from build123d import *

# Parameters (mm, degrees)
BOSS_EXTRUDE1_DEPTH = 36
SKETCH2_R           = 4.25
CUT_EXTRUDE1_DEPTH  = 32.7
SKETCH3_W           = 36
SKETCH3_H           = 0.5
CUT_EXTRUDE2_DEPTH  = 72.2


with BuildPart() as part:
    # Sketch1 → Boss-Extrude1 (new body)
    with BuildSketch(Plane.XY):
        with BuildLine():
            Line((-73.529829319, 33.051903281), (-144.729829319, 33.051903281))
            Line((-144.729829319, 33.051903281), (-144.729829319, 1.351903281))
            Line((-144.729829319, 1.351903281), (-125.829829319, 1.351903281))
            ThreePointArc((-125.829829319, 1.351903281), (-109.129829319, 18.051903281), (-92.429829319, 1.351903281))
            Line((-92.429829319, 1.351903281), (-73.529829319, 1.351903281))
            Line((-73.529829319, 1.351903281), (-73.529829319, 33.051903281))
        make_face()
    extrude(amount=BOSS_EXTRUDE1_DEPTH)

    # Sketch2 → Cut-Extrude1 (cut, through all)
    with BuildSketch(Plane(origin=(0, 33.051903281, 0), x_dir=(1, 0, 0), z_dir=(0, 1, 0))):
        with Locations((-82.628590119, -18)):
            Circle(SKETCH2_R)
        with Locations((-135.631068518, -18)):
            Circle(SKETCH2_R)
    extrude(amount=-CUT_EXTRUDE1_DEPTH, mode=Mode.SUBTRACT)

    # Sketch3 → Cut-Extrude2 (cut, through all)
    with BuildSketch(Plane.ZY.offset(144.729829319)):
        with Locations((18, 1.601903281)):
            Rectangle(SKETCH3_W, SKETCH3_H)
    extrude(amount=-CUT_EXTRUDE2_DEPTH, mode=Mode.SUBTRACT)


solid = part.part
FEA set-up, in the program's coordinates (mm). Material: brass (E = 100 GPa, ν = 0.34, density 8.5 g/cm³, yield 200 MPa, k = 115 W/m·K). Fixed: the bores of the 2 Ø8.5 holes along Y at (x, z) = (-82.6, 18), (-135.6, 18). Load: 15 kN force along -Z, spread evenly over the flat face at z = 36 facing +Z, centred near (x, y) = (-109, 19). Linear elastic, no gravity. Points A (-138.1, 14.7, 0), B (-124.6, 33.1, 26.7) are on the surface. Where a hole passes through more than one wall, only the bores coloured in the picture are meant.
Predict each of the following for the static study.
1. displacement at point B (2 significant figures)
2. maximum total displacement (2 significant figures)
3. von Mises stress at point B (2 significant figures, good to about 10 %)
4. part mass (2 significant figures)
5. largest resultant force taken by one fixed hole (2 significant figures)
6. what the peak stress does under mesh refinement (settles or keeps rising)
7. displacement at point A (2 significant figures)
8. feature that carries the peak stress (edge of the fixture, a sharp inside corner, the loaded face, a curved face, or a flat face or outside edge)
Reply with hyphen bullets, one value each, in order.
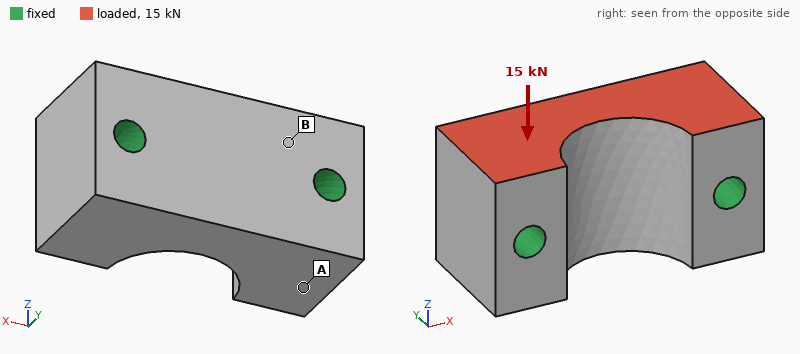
- 2.5 µm
- 4.7 µm
- 11 MPa
- 520 g
- 7.5 kN
- keeps rising
- 1.00 µm
- edge of the fixture
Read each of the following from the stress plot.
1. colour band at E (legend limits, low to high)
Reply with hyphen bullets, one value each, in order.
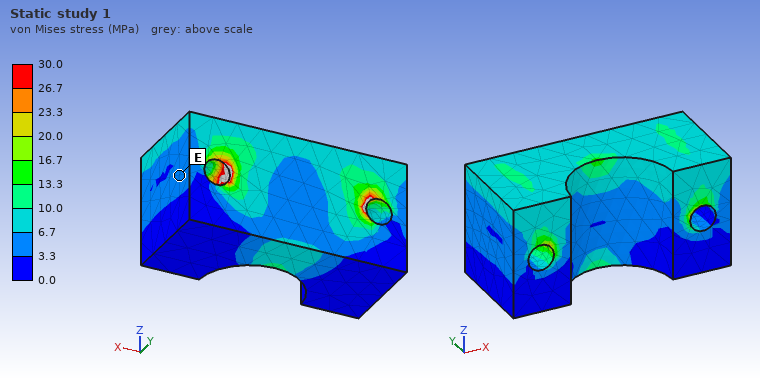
- 3.3 to 6.7 MPa
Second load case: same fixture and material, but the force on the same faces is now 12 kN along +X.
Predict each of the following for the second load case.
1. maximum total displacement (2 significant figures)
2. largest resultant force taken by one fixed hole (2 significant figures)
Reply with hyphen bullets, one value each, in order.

- 7.4 µm
- 6.6 kN
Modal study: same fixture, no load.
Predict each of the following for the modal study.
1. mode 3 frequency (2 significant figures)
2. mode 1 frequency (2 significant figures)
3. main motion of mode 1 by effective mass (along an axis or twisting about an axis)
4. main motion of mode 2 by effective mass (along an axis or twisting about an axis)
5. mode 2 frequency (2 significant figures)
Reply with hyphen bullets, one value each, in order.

- 20 kHz
- 15 kHz
- along Z
- along Y
- 17 kHz
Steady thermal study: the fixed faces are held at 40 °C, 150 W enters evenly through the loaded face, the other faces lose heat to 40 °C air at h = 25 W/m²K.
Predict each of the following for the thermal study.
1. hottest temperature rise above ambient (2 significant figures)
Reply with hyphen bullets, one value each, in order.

- 16 K
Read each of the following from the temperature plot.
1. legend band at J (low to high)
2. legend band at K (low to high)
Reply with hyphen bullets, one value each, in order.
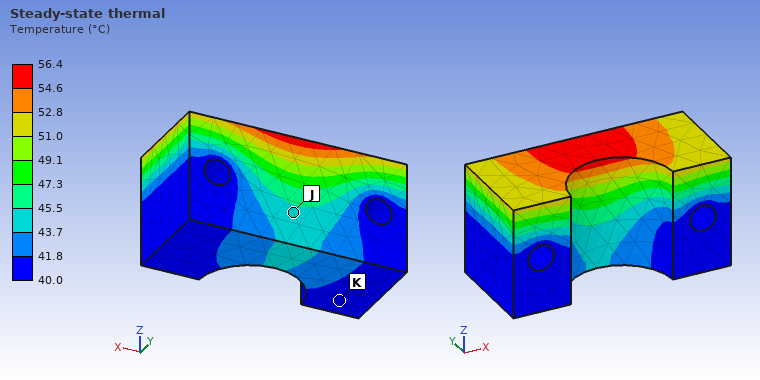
- 43.7 to 45.5 °C
- 40.0 to 41.8 °C
